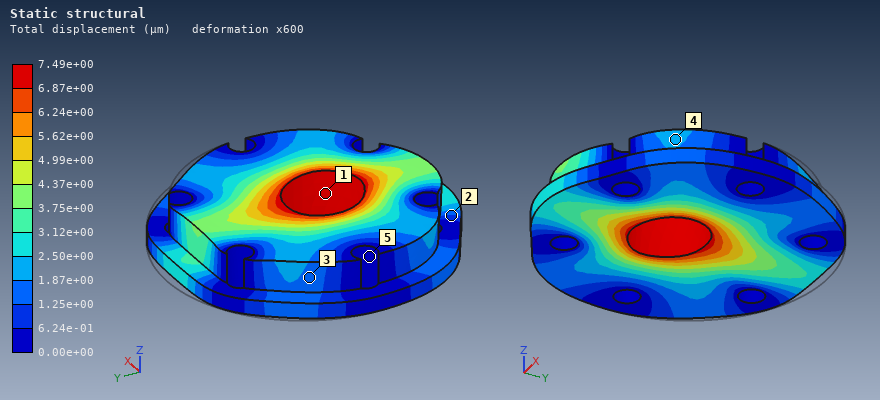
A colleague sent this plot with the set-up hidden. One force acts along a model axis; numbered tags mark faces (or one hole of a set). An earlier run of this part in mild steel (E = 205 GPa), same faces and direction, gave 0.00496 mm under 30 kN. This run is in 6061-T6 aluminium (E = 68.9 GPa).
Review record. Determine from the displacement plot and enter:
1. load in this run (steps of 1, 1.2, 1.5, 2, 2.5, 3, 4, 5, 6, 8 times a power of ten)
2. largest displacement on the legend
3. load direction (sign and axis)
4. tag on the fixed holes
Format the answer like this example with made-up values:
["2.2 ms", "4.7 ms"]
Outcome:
["15 kN", "7.49e+00 µm", "-Y", "5"]
